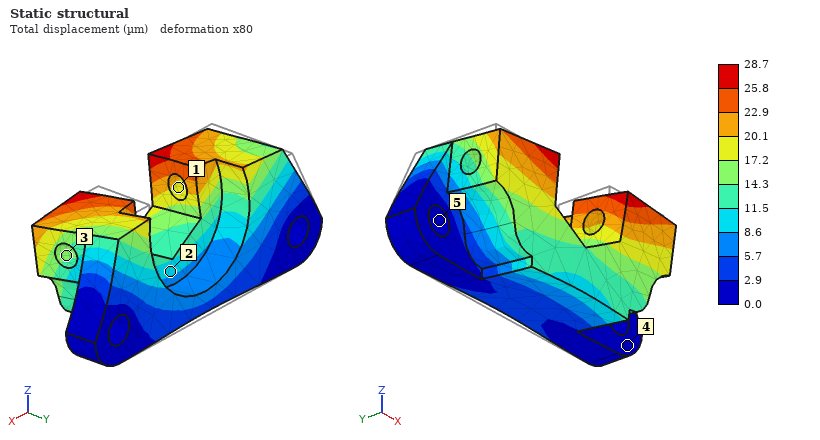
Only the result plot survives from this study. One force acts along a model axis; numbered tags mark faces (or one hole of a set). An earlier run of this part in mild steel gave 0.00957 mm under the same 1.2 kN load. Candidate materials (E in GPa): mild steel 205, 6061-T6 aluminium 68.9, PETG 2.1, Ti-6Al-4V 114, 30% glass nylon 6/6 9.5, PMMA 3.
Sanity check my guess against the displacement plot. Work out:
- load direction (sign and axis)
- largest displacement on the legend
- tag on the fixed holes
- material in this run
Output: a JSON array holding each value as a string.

["-Y", "28.7 µm", "5", "6061-T6 aluminium"]
